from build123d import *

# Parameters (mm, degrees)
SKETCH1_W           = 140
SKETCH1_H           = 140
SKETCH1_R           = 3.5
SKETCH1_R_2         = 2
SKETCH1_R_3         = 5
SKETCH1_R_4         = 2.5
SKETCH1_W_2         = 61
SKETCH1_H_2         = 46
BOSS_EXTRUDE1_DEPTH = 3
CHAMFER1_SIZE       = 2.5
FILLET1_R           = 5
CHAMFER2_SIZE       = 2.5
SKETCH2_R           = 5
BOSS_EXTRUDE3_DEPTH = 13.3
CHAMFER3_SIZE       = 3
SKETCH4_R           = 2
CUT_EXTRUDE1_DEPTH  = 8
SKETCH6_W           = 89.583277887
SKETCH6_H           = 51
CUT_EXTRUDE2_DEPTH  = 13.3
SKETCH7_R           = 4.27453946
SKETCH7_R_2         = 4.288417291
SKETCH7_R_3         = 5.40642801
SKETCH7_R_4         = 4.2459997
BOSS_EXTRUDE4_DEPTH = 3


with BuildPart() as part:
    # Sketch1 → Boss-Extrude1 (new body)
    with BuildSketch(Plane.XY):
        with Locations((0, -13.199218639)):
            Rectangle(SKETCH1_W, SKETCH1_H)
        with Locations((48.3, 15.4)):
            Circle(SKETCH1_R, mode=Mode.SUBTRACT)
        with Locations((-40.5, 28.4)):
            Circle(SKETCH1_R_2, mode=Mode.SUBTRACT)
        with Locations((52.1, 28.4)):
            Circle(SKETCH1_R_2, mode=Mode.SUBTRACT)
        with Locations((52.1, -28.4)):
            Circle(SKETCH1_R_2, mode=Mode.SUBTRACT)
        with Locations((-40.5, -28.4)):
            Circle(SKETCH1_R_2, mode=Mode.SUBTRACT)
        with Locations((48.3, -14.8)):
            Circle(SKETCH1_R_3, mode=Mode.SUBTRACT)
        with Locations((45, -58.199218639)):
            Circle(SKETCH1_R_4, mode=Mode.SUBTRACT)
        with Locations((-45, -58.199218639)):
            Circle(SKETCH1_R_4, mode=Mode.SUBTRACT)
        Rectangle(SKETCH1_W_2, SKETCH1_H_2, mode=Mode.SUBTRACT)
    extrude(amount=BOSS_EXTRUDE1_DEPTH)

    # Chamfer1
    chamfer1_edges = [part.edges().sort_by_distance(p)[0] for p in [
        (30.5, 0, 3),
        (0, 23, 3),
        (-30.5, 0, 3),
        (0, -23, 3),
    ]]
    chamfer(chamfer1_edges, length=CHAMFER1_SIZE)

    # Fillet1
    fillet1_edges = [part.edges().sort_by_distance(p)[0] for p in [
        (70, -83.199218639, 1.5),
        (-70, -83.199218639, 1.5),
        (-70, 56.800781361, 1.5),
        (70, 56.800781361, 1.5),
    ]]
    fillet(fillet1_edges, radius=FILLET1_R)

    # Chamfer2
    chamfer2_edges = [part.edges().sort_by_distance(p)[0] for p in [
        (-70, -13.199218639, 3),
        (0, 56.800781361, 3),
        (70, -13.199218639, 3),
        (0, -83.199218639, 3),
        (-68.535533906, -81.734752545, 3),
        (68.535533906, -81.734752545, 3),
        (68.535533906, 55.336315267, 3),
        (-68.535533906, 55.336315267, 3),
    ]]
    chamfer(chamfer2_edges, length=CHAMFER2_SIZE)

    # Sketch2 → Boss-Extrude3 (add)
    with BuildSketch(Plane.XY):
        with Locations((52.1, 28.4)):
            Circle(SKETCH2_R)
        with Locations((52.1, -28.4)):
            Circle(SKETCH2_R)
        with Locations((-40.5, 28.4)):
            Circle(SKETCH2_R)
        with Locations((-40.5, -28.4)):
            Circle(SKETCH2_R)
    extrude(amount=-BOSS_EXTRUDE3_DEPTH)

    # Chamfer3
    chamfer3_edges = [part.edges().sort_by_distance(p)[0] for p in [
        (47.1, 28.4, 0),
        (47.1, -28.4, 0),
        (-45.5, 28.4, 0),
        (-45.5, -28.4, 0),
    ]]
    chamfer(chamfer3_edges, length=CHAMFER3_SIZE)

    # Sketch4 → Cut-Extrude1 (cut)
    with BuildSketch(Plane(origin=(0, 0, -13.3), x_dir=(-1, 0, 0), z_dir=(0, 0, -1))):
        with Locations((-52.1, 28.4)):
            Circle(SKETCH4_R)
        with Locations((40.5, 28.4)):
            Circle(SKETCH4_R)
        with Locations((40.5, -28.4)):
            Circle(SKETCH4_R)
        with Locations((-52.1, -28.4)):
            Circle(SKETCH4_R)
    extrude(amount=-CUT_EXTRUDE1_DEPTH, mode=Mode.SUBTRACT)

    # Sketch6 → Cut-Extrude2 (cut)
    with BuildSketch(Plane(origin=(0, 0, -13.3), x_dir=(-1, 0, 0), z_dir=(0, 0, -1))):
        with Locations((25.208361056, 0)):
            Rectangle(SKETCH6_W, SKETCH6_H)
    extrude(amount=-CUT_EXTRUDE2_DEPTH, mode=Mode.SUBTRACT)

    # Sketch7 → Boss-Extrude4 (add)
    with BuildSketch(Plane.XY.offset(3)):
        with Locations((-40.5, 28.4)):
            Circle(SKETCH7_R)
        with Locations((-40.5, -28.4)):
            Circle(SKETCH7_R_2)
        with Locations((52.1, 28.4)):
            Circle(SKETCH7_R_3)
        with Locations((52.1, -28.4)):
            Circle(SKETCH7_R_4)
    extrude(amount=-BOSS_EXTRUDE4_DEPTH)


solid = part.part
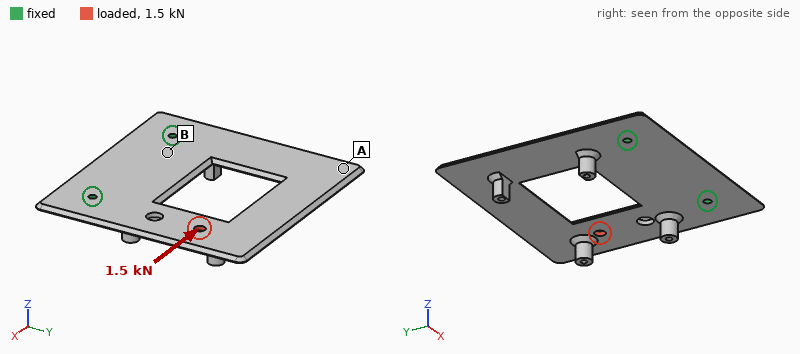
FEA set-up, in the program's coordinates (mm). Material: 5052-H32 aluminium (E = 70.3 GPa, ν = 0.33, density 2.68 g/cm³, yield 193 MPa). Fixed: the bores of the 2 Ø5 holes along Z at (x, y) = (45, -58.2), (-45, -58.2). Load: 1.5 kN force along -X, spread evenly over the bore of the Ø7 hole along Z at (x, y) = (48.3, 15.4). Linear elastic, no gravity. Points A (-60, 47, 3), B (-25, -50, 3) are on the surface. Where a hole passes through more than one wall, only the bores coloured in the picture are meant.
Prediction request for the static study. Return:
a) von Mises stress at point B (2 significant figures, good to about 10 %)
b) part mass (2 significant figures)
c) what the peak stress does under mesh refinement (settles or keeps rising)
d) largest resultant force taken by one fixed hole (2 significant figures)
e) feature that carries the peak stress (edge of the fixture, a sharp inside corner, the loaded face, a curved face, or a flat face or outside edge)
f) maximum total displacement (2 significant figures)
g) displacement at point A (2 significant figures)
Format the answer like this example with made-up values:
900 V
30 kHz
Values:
14 MPa
140 g
keeps rising
1.4 kN
a sharp inside corner
91 µm
83 µm
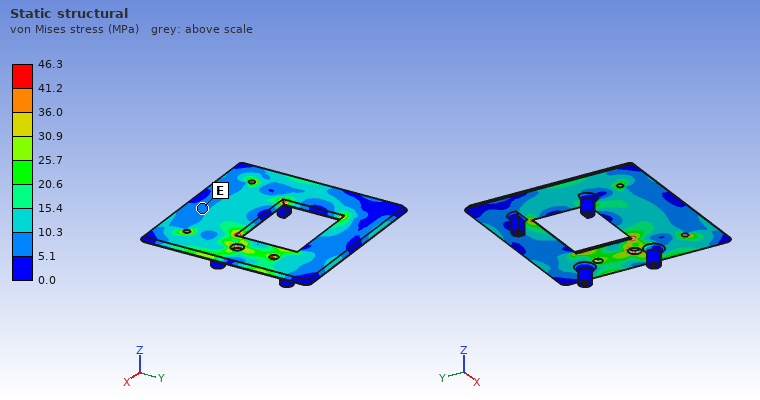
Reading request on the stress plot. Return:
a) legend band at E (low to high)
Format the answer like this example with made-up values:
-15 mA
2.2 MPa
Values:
5.1 to 10.3 MPa
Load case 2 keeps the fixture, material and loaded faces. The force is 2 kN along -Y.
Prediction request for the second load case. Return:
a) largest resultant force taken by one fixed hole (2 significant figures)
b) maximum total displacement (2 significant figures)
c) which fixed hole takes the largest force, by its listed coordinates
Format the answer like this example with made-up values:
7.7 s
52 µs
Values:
2.1 kN
58 µm
(45, -58.2)
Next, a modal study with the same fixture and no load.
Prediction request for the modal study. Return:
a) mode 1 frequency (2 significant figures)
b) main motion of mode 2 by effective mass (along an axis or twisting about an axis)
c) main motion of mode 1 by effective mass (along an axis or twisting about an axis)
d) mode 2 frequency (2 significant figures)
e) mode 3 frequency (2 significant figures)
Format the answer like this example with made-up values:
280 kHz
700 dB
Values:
160 Hz
twisting about Y
along Z
350 Hz
910 Hz
